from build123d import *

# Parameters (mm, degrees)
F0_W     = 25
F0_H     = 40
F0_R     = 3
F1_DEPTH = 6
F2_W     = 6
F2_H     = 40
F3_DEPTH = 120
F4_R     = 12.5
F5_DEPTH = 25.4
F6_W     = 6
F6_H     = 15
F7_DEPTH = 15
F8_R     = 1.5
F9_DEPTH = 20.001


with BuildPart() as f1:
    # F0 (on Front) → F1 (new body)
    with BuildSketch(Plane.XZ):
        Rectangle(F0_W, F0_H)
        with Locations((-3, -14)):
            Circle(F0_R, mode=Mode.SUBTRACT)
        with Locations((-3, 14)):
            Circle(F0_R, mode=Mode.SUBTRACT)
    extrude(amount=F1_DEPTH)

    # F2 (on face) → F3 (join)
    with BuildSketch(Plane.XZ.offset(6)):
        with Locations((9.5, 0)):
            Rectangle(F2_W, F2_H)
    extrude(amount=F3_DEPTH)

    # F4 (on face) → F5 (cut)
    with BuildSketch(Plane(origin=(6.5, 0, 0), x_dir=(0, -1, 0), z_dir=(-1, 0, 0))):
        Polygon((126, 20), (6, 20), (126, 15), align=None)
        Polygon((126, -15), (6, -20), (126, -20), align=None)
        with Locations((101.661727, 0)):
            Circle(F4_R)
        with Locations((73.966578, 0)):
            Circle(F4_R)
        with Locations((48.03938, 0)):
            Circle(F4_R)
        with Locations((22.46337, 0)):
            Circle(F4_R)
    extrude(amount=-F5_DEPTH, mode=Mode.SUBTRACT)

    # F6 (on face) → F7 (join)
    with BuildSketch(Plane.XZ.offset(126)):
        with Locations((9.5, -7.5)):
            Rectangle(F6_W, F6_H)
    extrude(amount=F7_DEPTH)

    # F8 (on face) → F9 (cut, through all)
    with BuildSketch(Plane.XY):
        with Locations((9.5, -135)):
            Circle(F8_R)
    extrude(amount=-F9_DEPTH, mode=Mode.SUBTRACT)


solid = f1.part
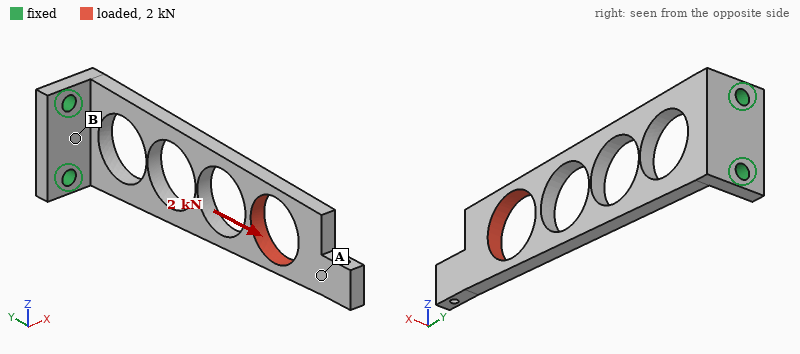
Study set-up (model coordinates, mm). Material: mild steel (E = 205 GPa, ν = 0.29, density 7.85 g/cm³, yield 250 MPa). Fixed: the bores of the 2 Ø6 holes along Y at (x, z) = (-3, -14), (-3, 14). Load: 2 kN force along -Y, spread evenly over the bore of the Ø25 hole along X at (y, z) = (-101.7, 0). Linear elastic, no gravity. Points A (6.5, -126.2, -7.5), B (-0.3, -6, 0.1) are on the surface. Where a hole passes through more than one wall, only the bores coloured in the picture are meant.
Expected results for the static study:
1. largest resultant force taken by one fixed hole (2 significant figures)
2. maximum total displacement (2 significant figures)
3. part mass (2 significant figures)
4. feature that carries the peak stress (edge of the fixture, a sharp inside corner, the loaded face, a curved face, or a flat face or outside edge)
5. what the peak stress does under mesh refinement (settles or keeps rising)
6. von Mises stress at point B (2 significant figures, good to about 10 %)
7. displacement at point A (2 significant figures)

1.0 kN
0.14 mm
160 g
edge of the fixture
keeps rising
27 MPa
0.12 mm
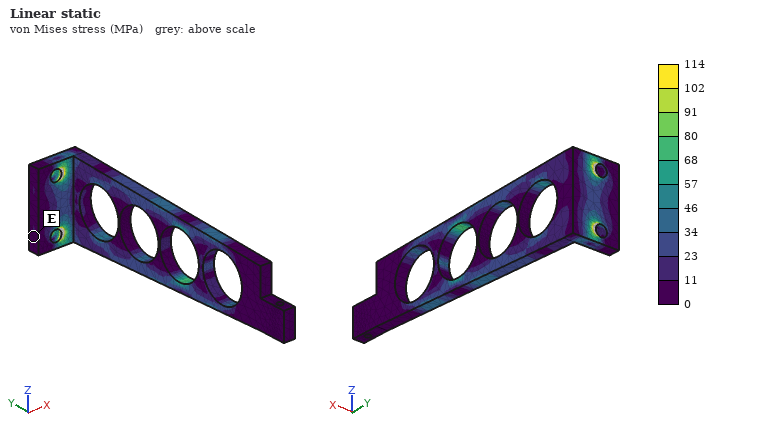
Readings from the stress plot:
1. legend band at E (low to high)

0 to 11 MPa
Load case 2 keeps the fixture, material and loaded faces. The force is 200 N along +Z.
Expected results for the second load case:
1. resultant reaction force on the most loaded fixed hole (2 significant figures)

650 N
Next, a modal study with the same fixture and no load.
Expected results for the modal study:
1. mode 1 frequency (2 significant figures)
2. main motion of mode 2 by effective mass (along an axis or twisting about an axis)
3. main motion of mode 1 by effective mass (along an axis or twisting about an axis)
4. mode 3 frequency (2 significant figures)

240 Hz
along Z
along X
1300 Hz
